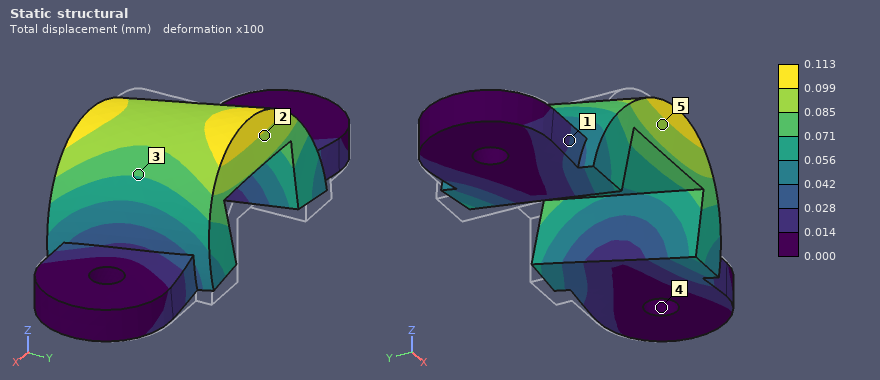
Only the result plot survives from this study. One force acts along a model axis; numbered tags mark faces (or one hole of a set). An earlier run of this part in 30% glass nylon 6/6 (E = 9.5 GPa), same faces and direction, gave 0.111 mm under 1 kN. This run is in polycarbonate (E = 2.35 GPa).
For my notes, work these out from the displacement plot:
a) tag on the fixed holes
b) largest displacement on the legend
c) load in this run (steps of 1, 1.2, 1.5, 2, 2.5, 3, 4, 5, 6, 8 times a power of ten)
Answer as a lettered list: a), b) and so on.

a) 4
b) 0.113 mm
c) 250 N
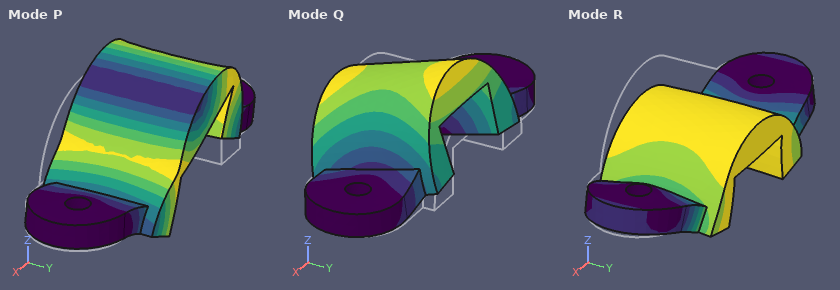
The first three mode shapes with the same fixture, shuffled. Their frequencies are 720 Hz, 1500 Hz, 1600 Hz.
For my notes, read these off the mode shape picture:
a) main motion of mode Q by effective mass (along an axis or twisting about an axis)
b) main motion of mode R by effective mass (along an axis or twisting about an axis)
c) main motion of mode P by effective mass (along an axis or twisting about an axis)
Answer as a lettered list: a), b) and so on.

a) along Y
b) along Z
c) along X
